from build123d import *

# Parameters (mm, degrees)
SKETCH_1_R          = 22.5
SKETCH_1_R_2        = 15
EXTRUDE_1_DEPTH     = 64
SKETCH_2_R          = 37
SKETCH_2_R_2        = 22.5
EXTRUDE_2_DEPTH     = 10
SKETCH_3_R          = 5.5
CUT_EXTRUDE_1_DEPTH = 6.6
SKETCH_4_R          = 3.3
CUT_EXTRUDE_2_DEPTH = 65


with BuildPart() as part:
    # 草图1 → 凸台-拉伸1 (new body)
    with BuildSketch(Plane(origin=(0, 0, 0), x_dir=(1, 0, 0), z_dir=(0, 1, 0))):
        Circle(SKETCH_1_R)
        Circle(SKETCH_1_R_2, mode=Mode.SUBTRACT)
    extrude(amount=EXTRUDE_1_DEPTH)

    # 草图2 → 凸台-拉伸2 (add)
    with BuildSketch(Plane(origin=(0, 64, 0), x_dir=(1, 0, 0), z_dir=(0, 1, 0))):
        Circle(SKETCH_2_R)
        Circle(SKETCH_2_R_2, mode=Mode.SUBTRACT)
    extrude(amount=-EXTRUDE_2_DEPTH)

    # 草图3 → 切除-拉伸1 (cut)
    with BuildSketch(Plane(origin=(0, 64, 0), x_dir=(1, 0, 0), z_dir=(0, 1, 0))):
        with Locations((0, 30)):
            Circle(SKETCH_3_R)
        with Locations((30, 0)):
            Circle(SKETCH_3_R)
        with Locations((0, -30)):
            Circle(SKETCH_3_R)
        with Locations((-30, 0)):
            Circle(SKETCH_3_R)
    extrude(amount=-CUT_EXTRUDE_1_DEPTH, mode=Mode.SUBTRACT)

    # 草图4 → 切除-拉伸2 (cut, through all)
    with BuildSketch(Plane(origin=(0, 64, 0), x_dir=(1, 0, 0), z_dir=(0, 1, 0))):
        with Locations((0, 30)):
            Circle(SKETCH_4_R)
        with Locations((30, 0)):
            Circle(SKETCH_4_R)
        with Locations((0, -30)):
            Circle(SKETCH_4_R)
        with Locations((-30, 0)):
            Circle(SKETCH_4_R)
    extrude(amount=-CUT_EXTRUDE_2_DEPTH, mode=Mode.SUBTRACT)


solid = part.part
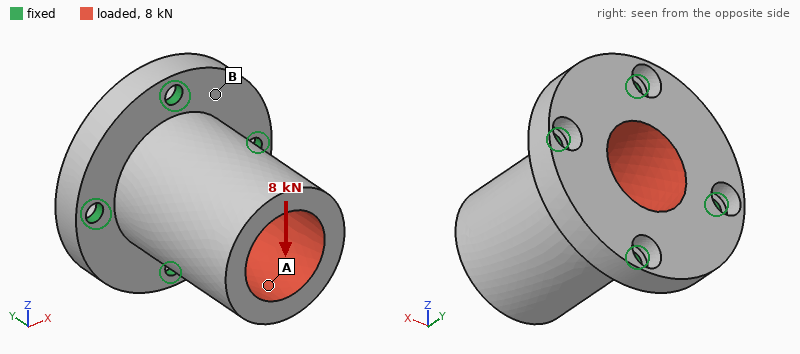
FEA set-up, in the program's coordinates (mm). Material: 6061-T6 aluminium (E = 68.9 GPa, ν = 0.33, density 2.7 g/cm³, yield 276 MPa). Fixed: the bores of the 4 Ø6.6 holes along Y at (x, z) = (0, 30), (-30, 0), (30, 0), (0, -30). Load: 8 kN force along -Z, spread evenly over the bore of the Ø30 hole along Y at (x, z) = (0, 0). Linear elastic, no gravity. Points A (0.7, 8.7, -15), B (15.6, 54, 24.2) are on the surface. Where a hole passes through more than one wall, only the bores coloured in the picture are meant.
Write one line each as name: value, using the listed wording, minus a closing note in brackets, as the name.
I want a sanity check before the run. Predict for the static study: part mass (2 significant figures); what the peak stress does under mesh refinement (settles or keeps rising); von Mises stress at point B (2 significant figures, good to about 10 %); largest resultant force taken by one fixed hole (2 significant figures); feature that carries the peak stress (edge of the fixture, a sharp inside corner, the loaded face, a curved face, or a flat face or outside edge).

part mass: 220 g
what the peak stress does under mesh refinement: keeps rising
von Mises stress at point B: 18 MPa
largest resultant force taken by one fixed hole: 3.6 kN
feature that carries the peak stress: edge of the fixture
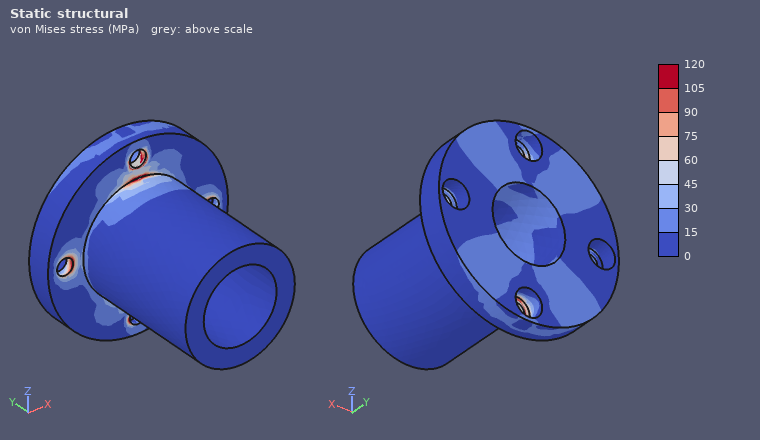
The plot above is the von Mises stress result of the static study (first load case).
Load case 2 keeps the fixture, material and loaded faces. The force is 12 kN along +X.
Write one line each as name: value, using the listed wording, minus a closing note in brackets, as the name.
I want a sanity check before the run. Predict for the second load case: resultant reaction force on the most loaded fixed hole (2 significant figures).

resultant reaction force on the most loaded fixed hole: 5.4 kN
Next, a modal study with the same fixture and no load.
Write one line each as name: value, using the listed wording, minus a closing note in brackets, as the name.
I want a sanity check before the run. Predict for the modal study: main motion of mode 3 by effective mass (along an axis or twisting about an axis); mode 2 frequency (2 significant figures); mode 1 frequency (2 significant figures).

main motion of mode 3 by effective mass: along Y
mode 2 frequency: 4800 Hz
mode 1 frequency: 4800 Hz
